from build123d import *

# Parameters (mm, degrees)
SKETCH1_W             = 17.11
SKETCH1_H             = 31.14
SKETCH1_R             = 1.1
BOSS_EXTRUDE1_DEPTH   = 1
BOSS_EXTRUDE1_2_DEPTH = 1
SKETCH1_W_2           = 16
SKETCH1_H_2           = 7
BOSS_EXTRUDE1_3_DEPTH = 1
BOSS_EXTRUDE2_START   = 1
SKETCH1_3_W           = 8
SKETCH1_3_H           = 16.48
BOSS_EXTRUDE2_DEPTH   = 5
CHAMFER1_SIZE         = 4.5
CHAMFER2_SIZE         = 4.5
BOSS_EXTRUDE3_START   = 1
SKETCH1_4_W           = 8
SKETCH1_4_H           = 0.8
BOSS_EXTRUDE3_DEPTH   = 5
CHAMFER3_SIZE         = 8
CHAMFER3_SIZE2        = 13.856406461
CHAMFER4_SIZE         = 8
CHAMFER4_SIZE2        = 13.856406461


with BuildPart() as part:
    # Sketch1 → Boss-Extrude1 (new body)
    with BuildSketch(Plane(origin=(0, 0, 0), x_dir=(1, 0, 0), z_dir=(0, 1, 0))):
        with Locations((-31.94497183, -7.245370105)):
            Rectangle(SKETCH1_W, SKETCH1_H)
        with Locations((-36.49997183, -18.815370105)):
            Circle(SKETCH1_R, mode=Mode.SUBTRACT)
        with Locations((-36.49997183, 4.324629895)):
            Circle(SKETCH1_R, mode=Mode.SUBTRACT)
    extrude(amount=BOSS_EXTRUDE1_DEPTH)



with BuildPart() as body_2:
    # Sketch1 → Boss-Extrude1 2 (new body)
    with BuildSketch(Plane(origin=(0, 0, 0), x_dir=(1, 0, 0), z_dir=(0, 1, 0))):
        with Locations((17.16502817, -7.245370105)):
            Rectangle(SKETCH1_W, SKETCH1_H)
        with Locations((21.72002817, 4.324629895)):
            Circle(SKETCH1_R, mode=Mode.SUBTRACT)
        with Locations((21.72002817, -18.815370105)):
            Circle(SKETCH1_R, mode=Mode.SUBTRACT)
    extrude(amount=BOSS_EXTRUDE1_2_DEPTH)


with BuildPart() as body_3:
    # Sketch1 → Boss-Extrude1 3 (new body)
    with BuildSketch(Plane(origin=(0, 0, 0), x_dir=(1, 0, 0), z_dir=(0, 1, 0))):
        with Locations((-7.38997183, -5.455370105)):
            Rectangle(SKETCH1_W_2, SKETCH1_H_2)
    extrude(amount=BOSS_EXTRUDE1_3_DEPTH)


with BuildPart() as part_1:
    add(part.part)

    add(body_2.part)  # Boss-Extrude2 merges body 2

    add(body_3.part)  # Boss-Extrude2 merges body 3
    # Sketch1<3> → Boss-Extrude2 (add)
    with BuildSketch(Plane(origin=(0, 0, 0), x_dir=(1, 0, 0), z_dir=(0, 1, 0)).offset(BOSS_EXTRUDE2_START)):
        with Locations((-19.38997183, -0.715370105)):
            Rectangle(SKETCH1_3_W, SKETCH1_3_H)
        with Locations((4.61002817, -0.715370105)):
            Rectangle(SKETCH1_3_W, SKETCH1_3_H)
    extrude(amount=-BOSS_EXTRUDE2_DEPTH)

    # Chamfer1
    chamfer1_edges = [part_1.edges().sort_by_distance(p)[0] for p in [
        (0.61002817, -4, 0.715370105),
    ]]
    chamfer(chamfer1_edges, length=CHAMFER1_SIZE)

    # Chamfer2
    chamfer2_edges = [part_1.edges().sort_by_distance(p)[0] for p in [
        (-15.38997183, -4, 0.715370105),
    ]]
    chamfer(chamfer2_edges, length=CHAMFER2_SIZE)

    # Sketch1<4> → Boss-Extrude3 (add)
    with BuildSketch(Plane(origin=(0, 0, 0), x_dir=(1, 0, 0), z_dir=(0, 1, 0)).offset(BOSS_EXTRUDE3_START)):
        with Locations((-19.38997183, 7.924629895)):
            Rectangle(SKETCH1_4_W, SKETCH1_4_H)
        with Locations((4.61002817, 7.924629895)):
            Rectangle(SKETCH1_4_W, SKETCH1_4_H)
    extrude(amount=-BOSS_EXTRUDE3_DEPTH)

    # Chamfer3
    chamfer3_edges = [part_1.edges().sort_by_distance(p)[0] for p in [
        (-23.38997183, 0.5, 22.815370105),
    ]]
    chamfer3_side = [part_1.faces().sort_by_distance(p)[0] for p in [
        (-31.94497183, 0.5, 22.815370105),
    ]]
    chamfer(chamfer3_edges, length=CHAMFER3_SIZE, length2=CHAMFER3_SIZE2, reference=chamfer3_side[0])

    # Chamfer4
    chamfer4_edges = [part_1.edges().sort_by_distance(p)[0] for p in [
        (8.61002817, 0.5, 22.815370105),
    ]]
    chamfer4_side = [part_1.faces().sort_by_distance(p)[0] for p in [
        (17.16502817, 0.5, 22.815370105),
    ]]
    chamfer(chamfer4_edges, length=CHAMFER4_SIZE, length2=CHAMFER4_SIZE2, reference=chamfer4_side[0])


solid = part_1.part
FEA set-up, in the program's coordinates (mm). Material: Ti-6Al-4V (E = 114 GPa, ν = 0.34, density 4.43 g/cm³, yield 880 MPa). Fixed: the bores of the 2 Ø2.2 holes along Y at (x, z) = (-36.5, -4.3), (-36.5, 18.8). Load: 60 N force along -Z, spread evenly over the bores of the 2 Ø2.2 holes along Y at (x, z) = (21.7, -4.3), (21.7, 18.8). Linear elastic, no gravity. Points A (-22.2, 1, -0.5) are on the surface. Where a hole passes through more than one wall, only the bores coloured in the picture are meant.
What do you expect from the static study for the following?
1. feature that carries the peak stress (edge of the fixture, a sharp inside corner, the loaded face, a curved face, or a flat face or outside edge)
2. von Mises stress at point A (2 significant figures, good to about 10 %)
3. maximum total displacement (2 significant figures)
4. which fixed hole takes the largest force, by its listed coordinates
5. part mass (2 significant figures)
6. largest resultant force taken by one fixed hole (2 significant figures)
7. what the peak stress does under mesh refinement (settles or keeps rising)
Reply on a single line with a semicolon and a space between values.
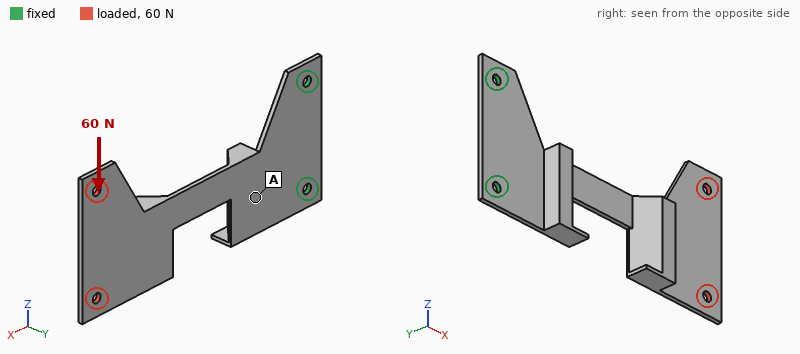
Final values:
a sharp inside corner; 37 MPa; 0.50 mm; (-36.5, 18.8); 9.3 g; 170 N; keeps rising
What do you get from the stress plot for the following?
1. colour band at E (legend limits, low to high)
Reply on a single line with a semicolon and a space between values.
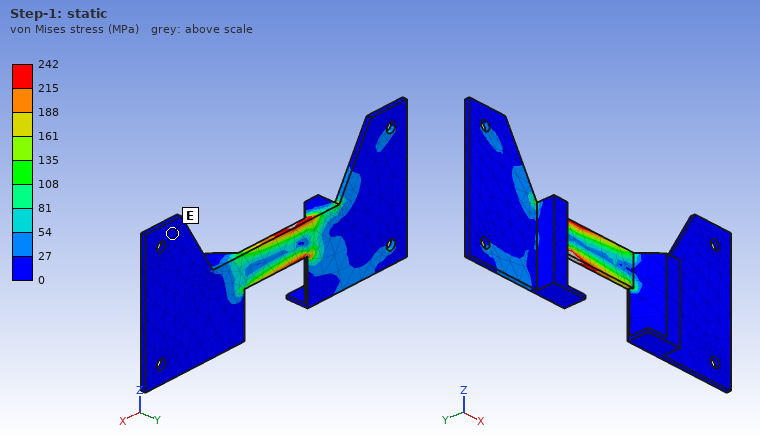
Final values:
0 to 27 MPa
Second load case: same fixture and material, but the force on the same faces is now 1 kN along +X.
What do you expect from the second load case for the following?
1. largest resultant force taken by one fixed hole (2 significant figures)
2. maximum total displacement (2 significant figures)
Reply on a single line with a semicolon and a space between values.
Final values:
570 N; 0.68 mm
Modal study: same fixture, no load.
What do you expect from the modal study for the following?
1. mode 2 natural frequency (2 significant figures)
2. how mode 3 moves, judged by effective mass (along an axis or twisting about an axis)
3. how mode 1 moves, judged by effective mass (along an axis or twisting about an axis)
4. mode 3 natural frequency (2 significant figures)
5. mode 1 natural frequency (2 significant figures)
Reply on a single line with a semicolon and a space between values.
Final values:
660 Hz; along Y; along Y; 1100 Hz; 160 Hz
